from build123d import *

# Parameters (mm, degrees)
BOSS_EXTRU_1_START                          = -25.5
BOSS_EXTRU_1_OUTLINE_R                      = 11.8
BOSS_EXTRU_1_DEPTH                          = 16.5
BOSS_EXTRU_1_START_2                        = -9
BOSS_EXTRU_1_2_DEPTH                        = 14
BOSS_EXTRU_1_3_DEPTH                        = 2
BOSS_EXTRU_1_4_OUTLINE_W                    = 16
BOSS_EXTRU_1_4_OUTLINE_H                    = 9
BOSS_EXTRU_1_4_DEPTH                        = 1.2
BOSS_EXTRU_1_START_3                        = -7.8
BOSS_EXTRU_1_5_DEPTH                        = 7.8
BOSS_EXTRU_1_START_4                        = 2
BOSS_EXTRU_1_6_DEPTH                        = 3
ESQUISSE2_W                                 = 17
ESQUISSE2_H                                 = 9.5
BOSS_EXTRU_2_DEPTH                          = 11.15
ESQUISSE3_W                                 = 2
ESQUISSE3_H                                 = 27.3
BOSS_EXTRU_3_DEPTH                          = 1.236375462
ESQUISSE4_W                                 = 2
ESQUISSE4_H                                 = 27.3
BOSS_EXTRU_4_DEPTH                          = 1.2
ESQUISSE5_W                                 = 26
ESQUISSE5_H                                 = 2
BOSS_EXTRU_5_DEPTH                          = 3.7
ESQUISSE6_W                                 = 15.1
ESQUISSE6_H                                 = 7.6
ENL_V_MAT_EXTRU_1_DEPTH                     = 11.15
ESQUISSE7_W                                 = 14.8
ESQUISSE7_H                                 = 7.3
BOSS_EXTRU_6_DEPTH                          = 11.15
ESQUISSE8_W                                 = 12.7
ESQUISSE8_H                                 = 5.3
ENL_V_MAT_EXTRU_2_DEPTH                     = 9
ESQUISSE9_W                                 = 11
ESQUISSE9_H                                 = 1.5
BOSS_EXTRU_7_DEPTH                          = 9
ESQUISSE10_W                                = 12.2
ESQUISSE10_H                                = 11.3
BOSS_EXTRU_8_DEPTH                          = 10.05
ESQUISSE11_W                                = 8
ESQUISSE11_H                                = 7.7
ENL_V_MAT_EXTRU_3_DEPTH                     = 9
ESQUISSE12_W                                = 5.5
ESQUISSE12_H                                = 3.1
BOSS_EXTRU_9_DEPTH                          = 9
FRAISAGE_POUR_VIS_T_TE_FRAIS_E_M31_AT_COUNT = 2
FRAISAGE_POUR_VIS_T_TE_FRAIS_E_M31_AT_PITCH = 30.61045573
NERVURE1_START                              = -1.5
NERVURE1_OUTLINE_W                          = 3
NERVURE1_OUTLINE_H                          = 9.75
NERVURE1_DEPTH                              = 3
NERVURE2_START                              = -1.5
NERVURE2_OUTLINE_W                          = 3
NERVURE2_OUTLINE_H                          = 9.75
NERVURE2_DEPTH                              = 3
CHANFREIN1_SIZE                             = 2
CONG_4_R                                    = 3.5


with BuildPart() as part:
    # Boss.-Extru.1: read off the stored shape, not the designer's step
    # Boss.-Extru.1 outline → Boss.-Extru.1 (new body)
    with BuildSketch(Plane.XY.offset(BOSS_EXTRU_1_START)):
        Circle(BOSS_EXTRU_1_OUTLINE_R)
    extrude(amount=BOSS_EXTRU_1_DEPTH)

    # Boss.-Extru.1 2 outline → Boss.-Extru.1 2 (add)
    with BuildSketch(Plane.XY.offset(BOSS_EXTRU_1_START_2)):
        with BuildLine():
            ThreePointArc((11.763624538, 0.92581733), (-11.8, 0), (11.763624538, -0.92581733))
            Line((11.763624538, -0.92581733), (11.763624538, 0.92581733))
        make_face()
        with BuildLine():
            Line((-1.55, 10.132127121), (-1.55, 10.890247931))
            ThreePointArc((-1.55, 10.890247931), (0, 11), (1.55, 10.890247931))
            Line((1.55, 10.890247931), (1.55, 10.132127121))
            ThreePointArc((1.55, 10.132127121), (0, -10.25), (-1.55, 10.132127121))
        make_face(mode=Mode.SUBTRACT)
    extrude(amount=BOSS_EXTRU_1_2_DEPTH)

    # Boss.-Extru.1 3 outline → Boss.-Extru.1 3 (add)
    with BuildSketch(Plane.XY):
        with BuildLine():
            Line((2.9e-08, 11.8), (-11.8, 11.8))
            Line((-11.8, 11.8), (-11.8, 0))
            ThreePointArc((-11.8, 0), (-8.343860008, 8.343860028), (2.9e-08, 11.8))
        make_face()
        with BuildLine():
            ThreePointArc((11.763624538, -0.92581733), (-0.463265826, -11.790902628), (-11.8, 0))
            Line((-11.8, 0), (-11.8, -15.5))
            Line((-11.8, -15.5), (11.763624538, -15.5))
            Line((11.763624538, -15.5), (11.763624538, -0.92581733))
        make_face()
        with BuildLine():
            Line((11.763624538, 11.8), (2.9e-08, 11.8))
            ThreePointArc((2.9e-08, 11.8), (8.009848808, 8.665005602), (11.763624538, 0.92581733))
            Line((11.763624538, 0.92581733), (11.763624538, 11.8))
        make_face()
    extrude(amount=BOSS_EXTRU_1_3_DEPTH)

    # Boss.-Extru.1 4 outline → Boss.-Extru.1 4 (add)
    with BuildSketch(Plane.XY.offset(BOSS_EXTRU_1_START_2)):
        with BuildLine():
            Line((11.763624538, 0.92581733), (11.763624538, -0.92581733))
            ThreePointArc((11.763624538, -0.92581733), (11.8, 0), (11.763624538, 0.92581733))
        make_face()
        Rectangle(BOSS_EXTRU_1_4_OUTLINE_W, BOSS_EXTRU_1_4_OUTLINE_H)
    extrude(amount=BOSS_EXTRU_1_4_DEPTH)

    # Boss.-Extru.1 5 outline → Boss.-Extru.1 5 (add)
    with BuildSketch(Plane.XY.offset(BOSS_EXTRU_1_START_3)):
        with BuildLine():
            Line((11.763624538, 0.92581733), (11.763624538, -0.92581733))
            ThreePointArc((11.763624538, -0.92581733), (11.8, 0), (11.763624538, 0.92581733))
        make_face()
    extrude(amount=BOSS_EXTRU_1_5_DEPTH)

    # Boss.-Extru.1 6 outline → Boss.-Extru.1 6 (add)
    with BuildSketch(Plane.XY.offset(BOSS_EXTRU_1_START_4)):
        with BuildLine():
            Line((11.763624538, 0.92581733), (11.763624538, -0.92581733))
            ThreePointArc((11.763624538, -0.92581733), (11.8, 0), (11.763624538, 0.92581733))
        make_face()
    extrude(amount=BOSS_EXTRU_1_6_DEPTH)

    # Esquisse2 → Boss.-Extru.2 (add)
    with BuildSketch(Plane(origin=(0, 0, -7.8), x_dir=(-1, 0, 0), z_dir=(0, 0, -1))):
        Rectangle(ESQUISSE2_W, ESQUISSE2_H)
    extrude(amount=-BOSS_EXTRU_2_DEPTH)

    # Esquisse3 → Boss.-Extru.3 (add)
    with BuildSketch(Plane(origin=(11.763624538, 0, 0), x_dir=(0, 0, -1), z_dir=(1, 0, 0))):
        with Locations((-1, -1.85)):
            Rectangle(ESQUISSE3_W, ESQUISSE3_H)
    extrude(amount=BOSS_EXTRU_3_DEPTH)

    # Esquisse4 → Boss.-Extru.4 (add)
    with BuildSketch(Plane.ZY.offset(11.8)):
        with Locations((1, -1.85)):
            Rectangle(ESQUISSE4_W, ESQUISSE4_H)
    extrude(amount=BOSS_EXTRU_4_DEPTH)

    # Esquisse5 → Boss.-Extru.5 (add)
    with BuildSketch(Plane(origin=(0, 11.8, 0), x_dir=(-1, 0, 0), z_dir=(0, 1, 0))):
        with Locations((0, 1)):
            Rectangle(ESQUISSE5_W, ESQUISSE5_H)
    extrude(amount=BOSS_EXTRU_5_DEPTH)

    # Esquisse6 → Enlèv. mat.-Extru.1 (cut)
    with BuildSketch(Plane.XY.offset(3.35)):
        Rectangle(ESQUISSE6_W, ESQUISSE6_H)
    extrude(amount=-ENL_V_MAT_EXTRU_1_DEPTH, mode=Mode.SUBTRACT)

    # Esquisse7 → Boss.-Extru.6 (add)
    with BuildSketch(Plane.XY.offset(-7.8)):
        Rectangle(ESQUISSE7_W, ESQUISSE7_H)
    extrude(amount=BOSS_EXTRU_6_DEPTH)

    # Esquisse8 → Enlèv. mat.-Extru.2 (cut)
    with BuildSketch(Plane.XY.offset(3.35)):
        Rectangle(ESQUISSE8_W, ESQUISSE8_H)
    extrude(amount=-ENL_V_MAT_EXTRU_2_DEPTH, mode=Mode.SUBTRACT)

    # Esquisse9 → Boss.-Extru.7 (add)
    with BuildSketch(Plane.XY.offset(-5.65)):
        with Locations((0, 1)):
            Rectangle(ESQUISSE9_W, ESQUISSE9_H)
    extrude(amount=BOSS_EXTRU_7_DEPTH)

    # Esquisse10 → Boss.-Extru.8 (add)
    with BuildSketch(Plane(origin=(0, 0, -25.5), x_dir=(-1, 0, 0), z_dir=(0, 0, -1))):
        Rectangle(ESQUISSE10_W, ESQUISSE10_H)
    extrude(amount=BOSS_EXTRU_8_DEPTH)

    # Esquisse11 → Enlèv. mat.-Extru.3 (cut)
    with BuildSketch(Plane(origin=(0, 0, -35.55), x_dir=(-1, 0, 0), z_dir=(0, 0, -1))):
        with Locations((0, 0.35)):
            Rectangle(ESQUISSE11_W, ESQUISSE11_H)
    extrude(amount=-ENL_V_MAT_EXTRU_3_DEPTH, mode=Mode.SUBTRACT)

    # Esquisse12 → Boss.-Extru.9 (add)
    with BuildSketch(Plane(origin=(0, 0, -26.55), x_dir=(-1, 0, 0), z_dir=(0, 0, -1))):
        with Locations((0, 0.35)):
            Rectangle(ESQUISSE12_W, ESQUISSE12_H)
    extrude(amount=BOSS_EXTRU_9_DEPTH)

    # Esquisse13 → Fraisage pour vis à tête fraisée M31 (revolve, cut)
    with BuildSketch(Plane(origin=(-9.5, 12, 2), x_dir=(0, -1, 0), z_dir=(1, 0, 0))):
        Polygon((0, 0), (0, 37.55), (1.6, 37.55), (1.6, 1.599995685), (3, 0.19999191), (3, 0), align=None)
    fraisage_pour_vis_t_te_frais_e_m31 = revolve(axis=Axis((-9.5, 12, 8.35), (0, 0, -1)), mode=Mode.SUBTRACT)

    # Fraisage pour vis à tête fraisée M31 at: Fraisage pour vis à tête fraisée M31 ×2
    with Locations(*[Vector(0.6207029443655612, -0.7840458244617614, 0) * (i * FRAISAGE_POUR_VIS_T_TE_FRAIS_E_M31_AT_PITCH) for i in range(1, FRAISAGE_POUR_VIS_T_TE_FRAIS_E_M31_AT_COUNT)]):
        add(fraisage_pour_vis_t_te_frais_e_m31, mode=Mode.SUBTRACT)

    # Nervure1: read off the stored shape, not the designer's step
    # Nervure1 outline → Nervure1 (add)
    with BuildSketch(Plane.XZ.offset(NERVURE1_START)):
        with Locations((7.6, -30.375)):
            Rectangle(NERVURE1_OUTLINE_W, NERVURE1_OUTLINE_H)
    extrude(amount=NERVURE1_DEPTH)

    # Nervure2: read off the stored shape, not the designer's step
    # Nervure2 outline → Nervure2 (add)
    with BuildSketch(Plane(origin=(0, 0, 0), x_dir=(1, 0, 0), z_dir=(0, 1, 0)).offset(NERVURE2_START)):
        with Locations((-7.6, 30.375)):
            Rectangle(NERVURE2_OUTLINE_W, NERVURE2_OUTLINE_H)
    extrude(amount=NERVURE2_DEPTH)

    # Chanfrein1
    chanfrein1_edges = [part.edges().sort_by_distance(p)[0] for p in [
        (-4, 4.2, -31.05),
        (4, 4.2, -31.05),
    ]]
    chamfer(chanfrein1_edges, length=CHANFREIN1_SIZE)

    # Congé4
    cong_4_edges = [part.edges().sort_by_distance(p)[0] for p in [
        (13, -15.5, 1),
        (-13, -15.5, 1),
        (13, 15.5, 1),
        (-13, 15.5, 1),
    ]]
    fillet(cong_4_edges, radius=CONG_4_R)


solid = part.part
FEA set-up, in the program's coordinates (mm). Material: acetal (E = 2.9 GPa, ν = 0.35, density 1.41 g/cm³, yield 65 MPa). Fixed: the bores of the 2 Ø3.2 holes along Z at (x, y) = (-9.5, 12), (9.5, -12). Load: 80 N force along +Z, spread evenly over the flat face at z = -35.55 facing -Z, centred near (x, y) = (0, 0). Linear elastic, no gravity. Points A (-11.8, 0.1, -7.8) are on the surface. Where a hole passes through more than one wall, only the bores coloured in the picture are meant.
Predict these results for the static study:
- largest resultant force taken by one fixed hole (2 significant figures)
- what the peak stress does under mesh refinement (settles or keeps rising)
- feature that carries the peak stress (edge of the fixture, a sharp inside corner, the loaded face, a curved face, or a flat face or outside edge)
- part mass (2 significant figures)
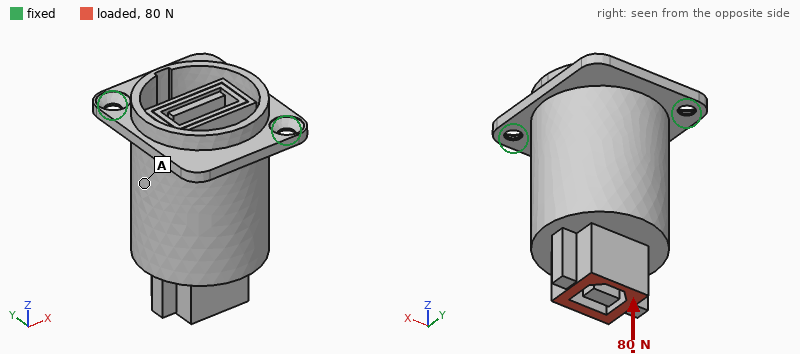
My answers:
40 N
keeps rising
edge of the fixture
17 g
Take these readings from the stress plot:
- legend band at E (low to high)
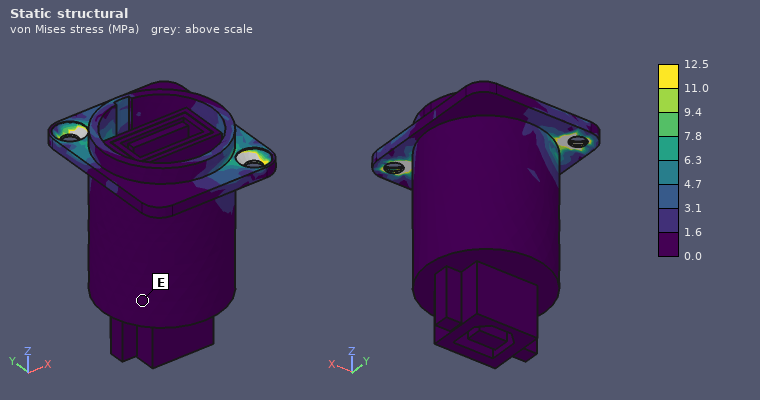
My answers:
0.0 to 1.6 MPa
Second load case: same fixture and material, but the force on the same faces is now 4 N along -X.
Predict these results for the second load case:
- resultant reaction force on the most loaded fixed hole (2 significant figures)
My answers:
3.8 N
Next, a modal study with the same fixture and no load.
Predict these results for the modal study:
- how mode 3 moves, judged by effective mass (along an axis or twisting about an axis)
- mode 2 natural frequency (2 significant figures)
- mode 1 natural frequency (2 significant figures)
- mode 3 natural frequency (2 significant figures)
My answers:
along Z
920 Hz
180 Hz
1400 Hz
